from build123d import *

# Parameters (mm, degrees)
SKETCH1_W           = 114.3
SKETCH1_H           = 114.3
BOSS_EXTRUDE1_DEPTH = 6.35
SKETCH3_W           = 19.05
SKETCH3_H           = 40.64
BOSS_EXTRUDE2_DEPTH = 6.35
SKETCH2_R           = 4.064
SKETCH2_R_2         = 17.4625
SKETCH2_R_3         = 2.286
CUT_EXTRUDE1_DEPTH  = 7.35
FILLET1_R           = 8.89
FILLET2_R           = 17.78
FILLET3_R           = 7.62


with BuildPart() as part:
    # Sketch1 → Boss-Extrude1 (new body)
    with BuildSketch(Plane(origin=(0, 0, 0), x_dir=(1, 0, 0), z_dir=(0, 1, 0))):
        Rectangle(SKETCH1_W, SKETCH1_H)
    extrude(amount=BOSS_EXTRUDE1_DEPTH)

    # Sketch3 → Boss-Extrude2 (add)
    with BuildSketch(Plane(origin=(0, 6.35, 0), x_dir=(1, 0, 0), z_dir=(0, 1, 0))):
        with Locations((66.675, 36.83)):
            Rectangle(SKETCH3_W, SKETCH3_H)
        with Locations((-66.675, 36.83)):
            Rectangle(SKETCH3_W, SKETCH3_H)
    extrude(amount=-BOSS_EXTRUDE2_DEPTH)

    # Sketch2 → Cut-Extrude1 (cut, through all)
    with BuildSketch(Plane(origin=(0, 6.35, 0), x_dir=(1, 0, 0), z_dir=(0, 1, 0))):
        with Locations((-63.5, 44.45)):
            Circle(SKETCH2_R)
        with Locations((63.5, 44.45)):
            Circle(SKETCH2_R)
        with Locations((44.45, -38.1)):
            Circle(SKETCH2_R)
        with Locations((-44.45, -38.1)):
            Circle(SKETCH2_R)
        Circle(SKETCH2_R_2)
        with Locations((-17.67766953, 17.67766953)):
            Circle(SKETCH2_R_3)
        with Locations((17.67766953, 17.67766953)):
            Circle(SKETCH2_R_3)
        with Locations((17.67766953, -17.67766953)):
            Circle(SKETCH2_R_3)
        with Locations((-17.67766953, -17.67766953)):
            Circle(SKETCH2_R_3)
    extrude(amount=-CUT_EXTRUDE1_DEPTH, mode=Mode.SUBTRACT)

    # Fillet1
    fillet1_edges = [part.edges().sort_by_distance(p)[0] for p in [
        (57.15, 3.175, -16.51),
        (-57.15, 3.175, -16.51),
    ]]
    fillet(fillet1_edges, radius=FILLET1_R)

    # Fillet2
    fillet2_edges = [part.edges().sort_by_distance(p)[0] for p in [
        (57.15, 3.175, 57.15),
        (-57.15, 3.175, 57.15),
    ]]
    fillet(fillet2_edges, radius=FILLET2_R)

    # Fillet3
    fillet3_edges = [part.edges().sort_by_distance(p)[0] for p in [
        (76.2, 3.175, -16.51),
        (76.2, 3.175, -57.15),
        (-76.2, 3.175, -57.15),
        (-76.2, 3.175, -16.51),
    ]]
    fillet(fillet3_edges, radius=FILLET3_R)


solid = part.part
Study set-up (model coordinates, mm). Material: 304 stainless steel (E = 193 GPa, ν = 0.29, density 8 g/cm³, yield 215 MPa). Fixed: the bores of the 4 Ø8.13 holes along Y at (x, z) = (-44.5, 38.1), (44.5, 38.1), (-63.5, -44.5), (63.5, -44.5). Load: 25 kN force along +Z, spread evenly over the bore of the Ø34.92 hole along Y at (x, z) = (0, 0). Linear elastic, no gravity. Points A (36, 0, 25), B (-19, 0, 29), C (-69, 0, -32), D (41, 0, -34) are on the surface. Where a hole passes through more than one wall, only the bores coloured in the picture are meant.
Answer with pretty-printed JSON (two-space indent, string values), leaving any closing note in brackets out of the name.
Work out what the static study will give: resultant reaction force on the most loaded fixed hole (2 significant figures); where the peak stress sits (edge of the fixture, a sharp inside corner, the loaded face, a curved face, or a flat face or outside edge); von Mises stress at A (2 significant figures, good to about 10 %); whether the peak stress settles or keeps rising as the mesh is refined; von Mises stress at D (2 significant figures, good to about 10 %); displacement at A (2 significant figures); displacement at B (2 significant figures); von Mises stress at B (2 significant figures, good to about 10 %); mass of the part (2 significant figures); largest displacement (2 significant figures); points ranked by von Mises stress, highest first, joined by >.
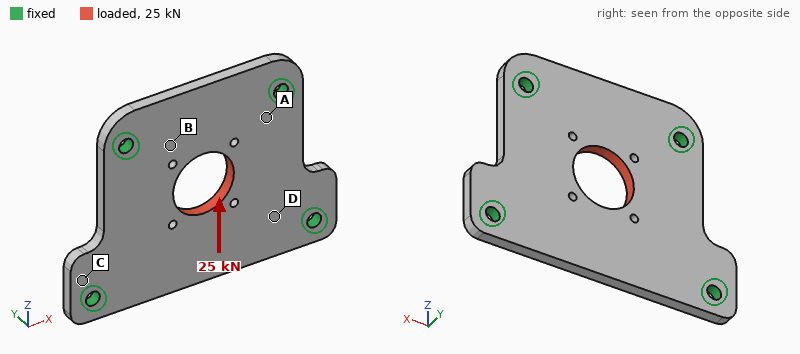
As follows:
{
  "resultant reaction force on the most loaded fixed hole": "9.1 kN",
  "where the peak stress sits": "edge of the fixture",
  "von Mises stress at A": "56 MPa",
  "whether the peak stress settles or keeps rising as the mesh is refined": "keeps rising",
  "von Mises stress at D": "25 MPa",
  "displacement at A": "4.5 µm",
  "displacement at B": "9.7 µm",
  "von Mises stress at B": "36 MPa",
  "mass of the part": "670 g",
  "largest displacement": "18 µm",
  "points ranked by von Mises stress, highest first, joined by >": "A > B > D > C"
}
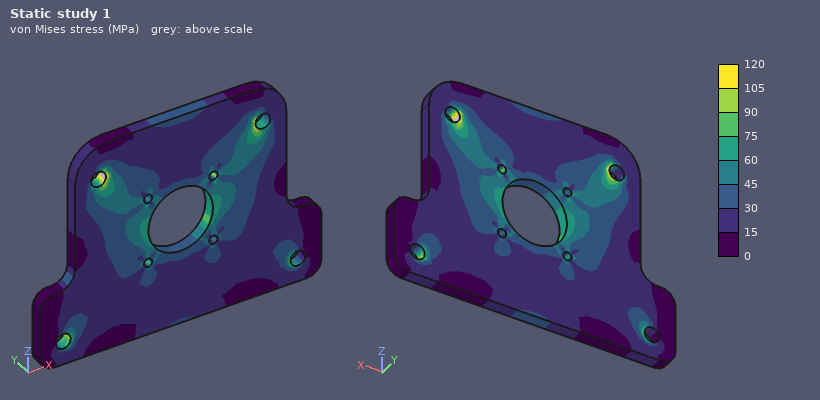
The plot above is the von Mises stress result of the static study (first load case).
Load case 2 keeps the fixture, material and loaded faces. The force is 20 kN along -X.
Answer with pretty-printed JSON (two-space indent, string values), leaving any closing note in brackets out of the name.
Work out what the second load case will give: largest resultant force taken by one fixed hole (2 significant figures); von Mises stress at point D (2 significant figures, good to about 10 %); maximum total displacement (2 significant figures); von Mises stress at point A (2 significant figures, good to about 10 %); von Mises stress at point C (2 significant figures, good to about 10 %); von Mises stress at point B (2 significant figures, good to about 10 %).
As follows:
{
  "largest resultant force taken by one fixed hole": "5.6 kN",
  "von Mises stress at point D": "25 MPa",
  "maximum total displacement": "9.9 µm",
  "von Mises stress at point A": "33 MPa",
  "von Mises stress at point C": "12 MPa",
  "von Mises stress at point B": "27 MPa"
}
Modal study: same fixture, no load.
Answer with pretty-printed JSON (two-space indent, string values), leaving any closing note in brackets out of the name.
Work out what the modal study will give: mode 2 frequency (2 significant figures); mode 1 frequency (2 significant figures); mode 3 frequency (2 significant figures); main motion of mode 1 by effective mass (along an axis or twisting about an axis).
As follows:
{
  "mode 2 frequency": "3700 Hz",
  "mode 1 frequency": "2100 Hz",
  "mode 3 frequency": "4400 Hz",
  "main motion of mode 1 by effective mass": "along Y"
}
